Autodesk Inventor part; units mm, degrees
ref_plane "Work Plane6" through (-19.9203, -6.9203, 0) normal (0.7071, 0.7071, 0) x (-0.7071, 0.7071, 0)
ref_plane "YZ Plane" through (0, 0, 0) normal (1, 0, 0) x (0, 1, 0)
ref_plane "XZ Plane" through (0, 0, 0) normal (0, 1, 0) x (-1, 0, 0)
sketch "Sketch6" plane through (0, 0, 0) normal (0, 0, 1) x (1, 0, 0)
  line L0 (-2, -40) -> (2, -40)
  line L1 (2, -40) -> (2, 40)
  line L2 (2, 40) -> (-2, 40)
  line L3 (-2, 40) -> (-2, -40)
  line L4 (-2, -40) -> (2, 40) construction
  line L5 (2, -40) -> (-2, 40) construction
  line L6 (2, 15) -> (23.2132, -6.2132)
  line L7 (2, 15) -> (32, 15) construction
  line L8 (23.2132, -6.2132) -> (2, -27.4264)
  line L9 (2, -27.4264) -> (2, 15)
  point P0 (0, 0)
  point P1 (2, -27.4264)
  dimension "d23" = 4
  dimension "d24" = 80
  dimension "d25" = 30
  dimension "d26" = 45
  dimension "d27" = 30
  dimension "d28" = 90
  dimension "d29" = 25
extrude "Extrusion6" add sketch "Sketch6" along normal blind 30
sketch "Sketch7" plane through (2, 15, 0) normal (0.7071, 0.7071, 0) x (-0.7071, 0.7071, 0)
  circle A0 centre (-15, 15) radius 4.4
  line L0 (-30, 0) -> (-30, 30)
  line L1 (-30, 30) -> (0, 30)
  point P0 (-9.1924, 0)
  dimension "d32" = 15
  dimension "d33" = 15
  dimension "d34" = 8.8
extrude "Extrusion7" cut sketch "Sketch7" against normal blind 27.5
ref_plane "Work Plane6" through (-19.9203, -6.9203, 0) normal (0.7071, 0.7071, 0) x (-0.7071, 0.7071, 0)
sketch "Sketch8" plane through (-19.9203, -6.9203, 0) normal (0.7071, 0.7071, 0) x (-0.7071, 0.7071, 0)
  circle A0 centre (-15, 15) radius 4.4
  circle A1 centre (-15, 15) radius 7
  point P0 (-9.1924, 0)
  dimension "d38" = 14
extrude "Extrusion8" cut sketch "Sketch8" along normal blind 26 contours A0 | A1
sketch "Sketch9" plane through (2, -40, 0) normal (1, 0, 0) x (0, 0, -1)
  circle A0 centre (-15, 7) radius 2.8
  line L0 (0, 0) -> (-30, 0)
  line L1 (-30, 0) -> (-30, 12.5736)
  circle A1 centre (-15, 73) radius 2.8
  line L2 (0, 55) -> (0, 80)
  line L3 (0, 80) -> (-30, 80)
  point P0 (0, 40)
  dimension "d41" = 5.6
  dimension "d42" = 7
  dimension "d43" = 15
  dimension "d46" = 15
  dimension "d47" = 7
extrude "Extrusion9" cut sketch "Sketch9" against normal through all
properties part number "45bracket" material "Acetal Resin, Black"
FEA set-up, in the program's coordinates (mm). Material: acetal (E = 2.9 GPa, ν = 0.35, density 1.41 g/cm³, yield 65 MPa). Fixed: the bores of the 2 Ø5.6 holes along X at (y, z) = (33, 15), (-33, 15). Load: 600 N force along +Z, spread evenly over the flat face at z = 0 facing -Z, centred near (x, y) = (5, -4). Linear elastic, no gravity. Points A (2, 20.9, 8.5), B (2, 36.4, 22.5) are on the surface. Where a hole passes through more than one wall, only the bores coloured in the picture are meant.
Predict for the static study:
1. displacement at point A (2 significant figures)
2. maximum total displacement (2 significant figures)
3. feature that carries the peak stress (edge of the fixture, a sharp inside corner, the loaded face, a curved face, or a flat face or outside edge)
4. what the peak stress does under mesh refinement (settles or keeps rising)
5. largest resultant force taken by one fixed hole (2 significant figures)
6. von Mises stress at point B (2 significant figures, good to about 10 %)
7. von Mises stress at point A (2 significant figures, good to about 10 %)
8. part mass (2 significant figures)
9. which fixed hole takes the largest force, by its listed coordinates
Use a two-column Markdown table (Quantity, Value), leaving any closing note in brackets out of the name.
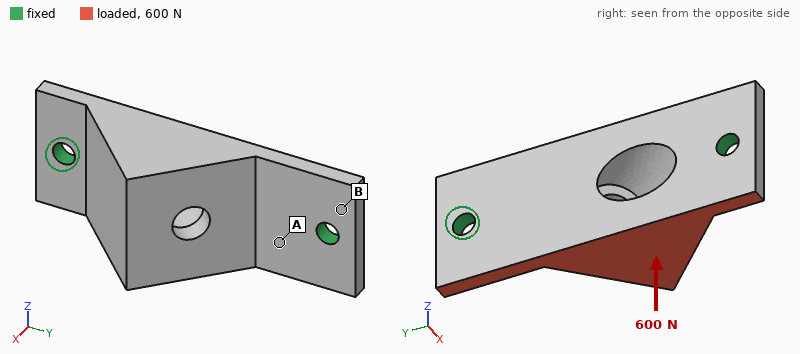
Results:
| Quantity | Value |
|---|---|
| displacement at point A | 0.12 mm |
| maximum total displacement | 0.67 mm |
| feature that carries the peak stress | edge of the fixture |
| what the peak stress does under mesh refinement | keeps rising |
| largest resultant force taken by one fixed hole | 340 N |
| von Mises stress at point B | 4.5 MPa |
| von Mises stress at point A | 9.6 MPa |
| part mass | 28 g |
| which fixed hole takes the largest force, by its listed coordinates | (-33, 15) |
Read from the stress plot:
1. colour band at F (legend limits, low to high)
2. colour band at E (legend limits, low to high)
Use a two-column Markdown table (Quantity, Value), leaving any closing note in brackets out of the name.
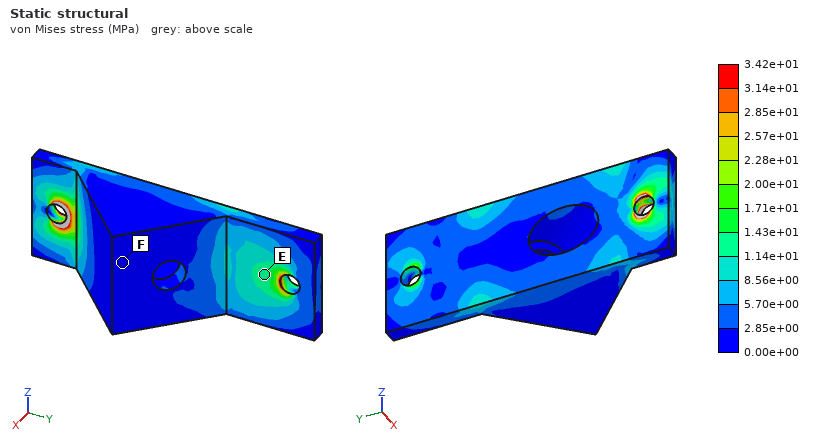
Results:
| Quantity | Value |
|---|---|
| colour band at F | 0.00e+00 to 2.85e+00 MPa |
| colour band at E | 1.14e+01 to 1.43e+01 MPa |
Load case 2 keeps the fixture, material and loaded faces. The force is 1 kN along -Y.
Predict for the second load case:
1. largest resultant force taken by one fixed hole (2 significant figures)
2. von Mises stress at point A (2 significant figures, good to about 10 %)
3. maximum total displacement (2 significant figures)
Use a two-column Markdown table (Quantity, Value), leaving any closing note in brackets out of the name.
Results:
| Quantity | Value |
|---|---|
| largest resultant force taken by one fixed hole | 580 N |
| von Mises stress at point A | 11 MPa |
| maximum total displacement | 0.17 mm |
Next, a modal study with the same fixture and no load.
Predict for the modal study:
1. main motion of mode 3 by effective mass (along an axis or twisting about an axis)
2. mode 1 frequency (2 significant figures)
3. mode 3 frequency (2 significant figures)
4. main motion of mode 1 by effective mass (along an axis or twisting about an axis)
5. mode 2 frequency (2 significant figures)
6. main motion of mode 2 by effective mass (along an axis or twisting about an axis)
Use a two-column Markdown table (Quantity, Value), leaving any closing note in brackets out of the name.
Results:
| Quantity | Value |
|---|---|
| main motion of mode 3 by effective mass | along Z |
| mode 1 frequency | 960 Hz |
| mode 3 frequency | 3300 Hz |
| main motion of mode 1 by effective mass | along Z |
| mode 2 frequency | 1400 Hz |
| main motion of mode 2 by effective mass | along X |
